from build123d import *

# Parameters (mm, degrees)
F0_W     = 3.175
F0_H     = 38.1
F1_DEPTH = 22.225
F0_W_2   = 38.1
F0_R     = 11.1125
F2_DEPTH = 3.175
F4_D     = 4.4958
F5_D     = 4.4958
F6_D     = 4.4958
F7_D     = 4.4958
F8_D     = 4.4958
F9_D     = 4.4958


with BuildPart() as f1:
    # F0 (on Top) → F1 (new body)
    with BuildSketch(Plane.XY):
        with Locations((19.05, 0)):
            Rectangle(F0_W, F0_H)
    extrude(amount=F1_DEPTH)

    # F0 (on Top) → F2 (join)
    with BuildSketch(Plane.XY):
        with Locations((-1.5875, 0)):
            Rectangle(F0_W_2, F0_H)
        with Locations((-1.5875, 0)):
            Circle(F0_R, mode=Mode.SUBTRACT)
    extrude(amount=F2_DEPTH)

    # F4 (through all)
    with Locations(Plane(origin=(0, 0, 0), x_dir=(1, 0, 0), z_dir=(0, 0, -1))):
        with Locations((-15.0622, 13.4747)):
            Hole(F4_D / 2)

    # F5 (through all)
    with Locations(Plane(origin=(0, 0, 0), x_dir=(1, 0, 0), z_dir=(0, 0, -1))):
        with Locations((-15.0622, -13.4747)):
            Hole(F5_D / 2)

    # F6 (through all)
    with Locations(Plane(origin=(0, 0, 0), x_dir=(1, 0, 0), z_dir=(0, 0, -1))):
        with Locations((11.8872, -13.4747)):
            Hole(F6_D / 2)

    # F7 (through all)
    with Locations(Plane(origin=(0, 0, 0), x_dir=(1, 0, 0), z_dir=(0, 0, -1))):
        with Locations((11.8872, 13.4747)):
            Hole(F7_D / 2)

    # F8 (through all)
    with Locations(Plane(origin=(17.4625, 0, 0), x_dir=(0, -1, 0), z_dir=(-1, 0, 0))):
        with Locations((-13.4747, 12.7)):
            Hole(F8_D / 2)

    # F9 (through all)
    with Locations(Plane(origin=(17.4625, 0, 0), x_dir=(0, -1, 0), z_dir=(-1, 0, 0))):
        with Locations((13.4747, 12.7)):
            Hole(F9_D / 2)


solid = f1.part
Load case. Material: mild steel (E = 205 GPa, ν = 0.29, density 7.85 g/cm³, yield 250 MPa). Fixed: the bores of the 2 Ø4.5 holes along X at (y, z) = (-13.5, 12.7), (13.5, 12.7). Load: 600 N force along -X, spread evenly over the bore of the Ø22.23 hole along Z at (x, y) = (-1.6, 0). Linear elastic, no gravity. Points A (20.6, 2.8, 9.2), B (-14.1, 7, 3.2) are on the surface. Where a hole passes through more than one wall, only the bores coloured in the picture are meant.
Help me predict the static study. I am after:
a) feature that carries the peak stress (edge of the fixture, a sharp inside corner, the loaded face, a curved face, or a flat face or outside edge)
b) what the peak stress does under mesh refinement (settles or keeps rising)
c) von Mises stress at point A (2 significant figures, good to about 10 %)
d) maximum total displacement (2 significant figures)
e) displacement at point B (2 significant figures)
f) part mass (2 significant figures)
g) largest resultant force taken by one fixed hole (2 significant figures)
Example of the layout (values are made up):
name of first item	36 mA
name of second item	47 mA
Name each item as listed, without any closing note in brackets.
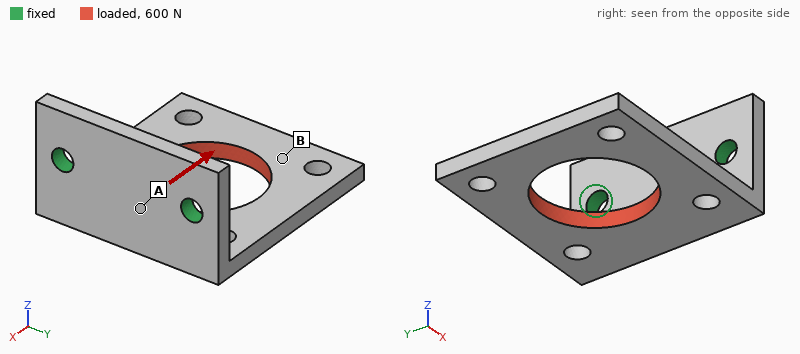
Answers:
feature that carries the peak stress	edge of the fixture
what the peak stress does under mesh refinement	keeps rising
von Mises stress at point A	32 MPa
maximum total displacement	67 µm
displacement at point B	55 µm
part mass	45 g
largest resultant force taken by one fixed hole	300 N
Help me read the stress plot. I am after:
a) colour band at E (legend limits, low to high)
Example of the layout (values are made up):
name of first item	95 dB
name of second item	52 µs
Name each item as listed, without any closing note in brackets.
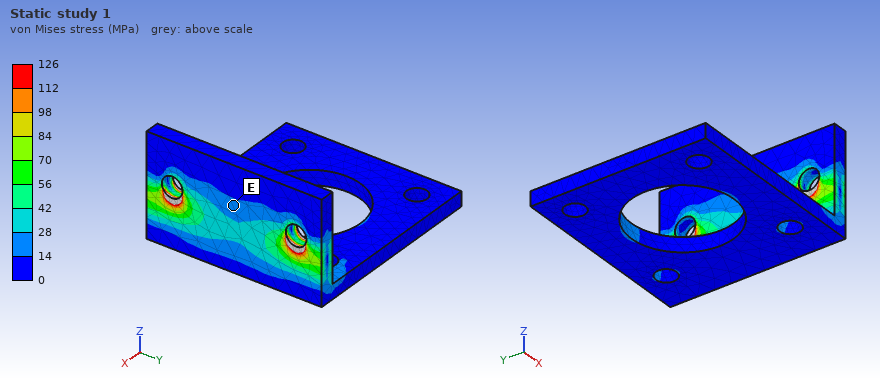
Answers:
colour band at E	14 to 28 MPa
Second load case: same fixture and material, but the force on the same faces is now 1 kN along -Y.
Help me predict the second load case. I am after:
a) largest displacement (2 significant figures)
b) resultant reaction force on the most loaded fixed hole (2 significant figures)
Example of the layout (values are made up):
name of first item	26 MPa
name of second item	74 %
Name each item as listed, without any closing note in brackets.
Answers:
largest displacement	86 µm
resultant reaction force on the most loaded fixed hole	950 N
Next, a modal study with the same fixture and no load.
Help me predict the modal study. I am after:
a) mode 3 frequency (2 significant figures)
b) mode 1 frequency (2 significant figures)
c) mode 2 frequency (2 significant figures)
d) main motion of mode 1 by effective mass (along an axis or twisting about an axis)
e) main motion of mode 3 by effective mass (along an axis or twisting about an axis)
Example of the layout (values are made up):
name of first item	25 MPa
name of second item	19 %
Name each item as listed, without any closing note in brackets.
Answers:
mode 3 frequency	4400 Hz
mode 1 frequency	1200 Hz
mode 2 frequency	3000 Hz
main motion of mode 1 by effective mass	along Z
main motion of mode 3 by effective mass	along Y
